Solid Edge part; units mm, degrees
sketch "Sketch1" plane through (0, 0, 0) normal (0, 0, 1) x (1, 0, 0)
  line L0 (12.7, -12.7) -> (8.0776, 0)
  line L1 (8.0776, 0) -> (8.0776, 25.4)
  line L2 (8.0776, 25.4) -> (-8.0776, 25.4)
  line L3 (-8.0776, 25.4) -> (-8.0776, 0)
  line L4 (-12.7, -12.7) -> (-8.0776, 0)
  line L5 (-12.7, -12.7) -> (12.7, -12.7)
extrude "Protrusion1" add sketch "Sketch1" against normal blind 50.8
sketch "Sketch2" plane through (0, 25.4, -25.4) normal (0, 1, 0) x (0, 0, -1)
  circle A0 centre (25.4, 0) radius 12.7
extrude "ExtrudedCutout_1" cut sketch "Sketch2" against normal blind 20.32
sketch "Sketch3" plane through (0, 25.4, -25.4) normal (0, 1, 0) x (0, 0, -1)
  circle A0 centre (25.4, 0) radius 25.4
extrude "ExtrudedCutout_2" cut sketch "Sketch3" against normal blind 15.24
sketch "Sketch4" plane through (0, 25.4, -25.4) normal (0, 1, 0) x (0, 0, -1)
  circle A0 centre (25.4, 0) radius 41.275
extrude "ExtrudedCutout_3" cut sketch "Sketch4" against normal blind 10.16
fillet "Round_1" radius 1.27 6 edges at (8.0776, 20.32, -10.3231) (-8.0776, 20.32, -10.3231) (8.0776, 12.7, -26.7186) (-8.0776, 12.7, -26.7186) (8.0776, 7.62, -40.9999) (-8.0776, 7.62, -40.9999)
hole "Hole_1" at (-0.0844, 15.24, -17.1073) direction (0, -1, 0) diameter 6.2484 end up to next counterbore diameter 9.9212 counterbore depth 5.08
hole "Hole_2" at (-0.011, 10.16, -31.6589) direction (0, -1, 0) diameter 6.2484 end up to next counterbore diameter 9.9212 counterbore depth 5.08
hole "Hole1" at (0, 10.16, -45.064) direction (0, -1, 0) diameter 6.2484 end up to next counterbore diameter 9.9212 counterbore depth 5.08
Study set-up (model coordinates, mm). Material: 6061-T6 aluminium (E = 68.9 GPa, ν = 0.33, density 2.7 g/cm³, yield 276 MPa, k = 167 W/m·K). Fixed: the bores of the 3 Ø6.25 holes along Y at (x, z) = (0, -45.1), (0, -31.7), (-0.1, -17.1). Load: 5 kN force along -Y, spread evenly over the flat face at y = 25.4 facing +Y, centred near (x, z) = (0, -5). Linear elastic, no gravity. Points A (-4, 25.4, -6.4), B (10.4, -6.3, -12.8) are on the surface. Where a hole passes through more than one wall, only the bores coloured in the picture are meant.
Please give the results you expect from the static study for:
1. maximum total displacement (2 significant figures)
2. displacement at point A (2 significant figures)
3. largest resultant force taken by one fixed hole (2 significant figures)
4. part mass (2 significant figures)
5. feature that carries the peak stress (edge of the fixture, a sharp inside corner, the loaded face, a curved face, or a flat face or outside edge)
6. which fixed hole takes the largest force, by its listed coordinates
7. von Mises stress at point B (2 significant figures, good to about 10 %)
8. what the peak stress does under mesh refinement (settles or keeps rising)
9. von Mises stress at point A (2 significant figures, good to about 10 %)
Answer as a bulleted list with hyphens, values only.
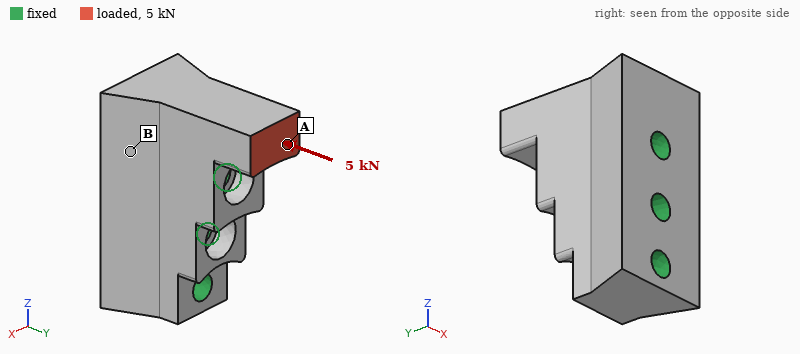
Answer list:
- 28 µm
- 23 µm
- 5.4 kN
- 59 g
- edge of the fixture
- (-0.1, -17.1)
- 9.0 MPa
- keeps rising
- 32 MPa
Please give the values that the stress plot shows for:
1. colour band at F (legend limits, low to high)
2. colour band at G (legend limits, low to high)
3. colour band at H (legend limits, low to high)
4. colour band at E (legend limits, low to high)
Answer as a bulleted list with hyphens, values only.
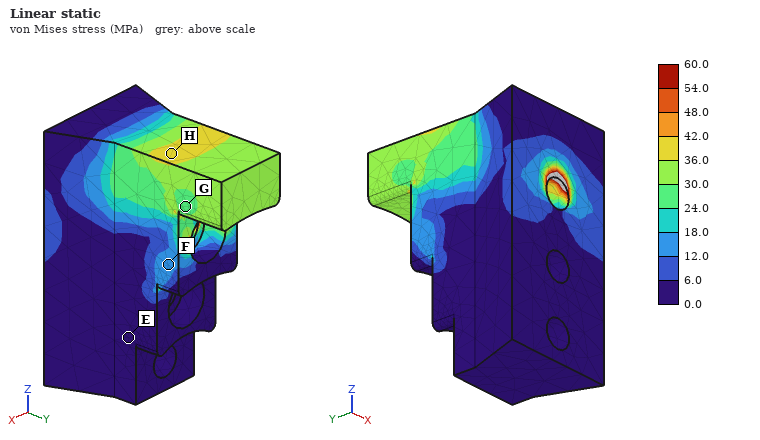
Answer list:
- 12.0 to 18.0 MPa
- 24.0 to 30.0 MPa
- 36.0 to 42.0 MPa
- 0.0 to 6.0 MPa
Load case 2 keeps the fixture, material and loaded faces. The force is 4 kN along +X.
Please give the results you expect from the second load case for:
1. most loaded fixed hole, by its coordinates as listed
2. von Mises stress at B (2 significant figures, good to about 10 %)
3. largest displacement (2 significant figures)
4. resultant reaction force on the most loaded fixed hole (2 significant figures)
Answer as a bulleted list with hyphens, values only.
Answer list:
- (-0.1, -17.1)
- 29 MPa
- 0.11 mm
- 5.1 kN
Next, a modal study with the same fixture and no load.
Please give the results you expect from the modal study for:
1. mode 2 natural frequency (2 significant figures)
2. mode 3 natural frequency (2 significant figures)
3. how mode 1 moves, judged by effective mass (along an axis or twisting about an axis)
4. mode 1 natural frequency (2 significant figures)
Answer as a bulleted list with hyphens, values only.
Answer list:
- 20 kHz
- 27 kHz
- along X
- 17 kHz
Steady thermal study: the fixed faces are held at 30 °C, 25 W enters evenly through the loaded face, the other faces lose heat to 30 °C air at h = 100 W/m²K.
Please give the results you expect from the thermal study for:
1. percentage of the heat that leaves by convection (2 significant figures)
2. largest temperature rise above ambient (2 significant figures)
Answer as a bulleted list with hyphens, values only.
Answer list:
- 5.4 %
- 19 K
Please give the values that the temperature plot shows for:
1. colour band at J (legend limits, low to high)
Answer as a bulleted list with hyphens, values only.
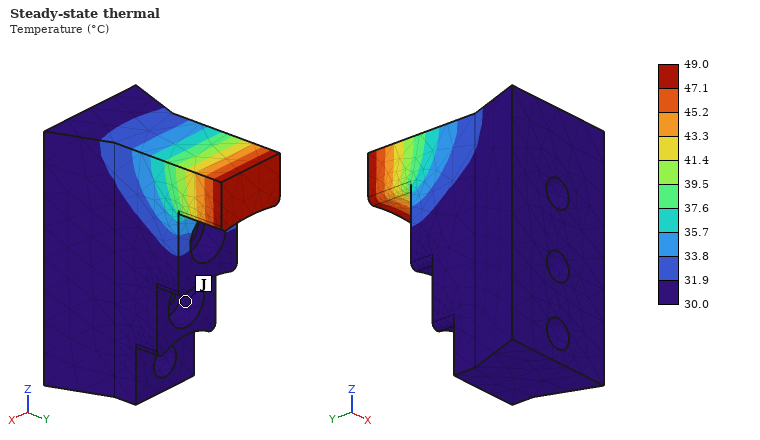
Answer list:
- 30.0 to 31.9 °C
